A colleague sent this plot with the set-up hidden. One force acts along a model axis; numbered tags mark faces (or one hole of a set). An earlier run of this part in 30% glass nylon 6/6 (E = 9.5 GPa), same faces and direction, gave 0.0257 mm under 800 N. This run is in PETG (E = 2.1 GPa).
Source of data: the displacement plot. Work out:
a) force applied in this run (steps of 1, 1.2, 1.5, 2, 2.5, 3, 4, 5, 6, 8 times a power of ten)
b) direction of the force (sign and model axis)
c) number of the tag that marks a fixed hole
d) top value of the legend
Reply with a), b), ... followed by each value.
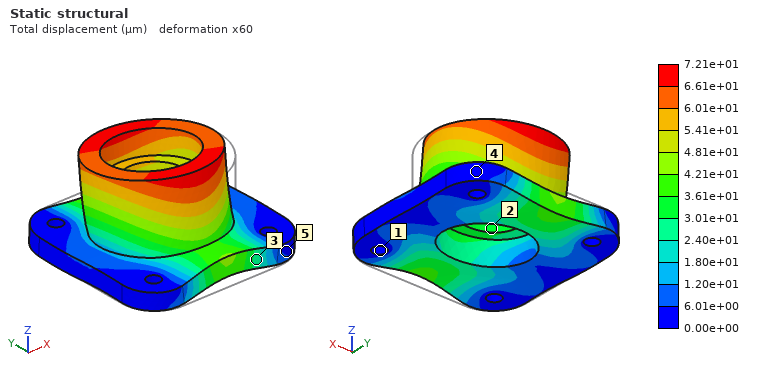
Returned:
a) 500 N
b) +Y
c) 1
d) 7.21e+01 µm
